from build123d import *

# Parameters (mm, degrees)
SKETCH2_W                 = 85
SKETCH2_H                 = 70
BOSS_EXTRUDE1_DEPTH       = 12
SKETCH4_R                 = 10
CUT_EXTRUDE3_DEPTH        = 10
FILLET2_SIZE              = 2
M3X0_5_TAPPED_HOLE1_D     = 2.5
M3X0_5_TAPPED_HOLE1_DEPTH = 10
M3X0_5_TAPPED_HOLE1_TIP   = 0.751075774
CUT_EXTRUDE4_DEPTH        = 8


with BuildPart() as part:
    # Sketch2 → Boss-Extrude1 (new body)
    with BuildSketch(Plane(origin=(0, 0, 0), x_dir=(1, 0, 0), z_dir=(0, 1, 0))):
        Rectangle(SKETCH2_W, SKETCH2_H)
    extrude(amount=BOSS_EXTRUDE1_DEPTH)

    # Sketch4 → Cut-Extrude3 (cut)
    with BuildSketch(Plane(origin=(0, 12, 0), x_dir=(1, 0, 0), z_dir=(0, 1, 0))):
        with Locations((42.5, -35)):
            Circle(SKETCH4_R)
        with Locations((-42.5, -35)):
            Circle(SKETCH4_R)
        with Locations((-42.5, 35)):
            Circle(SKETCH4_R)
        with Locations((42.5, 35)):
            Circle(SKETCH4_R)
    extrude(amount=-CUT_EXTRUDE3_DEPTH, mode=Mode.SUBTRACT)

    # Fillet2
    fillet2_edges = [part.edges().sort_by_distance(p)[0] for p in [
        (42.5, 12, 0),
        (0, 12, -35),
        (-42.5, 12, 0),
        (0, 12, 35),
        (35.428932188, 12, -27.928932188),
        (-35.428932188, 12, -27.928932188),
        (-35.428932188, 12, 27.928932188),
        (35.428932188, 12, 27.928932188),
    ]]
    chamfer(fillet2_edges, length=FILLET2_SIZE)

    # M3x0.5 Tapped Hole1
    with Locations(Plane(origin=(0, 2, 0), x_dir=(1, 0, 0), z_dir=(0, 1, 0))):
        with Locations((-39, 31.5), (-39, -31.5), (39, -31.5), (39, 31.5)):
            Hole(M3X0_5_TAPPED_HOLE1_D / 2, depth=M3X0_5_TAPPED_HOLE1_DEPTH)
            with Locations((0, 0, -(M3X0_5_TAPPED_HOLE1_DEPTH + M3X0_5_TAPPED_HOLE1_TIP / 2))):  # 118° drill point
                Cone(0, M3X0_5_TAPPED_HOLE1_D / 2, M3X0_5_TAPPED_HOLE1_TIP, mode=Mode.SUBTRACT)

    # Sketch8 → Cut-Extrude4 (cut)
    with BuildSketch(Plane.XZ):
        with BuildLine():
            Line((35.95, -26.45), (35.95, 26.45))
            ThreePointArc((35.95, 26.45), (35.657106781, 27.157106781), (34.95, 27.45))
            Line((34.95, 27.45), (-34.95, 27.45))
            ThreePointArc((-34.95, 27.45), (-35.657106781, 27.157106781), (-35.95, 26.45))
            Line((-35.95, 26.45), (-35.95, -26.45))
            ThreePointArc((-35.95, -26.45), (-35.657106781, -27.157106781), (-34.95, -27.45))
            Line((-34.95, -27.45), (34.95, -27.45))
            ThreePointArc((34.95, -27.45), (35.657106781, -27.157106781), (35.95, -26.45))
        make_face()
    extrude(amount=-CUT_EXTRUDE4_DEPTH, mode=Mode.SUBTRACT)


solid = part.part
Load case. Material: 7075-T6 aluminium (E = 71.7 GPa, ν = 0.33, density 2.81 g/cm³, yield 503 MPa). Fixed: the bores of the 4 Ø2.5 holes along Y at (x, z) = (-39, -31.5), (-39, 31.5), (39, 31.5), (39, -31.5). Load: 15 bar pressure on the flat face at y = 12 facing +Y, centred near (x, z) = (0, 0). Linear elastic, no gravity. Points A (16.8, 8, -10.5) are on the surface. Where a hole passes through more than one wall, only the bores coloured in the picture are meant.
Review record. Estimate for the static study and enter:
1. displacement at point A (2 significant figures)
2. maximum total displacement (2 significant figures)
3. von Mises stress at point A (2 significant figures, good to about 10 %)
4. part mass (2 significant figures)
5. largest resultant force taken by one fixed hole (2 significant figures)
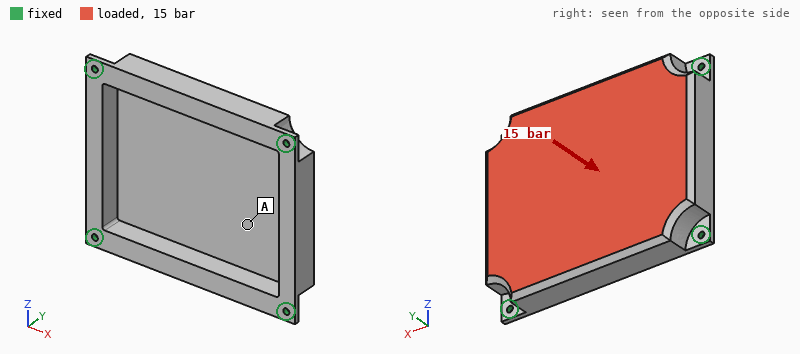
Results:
0.22 mm
0.29 mm
50 MPa
100 g
3.2 kN
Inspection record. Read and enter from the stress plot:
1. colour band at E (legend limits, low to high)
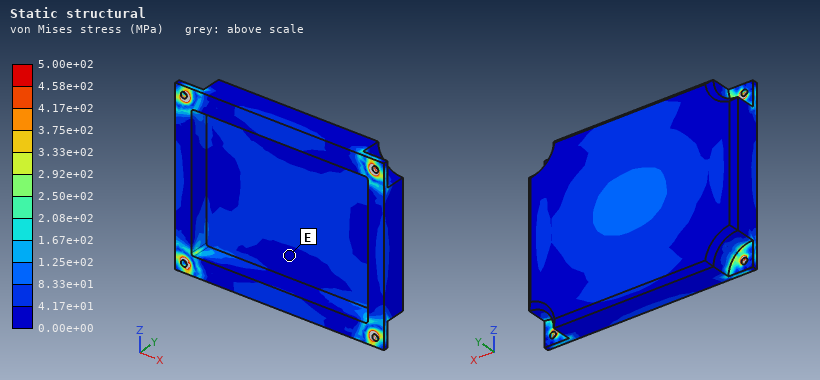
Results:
0.00e+00 to 4.17e+01 MPa
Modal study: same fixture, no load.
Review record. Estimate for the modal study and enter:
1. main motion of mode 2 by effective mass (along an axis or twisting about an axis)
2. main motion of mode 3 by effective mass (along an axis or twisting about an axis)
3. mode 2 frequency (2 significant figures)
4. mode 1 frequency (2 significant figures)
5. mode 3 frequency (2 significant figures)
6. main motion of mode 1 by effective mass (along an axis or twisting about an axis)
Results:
twisting about X
twisting about Z
5100 Hz
3800 Hz
6100 Hz
along Y
